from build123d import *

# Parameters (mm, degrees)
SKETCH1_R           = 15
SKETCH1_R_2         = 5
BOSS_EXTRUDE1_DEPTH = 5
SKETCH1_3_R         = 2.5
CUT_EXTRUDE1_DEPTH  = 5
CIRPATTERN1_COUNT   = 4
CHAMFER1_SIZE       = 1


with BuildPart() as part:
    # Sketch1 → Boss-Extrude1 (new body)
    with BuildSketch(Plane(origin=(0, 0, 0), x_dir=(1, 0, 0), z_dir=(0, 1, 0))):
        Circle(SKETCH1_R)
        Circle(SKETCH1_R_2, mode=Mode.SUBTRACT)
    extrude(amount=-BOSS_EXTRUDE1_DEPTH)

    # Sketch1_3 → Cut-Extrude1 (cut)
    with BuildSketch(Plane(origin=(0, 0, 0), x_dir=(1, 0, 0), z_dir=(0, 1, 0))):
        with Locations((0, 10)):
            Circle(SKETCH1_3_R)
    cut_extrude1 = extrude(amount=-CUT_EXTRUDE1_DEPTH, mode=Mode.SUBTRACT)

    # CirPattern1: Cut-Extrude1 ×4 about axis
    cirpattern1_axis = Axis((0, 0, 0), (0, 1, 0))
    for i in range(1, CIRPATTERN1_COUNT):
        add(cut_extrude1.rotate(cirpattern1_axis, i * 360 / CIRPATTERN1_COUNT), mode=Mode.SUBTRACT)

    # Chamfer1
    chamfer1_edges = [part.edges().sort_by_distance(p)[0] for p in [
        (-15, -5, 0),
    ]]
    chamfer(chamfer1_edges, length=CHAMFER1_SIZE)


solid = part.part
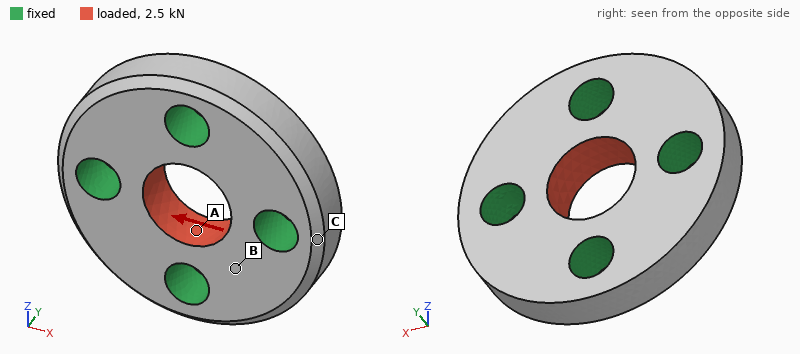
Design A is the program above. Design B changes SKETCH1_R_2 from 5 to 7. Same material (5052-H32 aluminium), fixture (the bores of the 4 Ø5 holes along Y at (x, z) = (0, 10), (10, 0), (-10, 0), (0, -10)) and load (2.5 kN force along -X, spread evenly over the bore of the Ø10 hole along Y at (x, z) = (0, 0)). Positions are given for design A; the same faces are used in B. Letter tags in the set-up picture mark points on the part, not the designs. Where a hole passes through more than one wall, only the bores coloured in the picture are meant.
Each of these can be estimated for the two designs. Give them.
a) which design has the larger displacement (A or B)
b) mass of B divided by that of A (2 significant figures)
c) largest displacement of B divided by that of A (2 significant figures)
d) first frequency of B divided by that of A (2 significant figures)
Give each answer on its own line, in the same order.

A
0.86
0.75
0.98
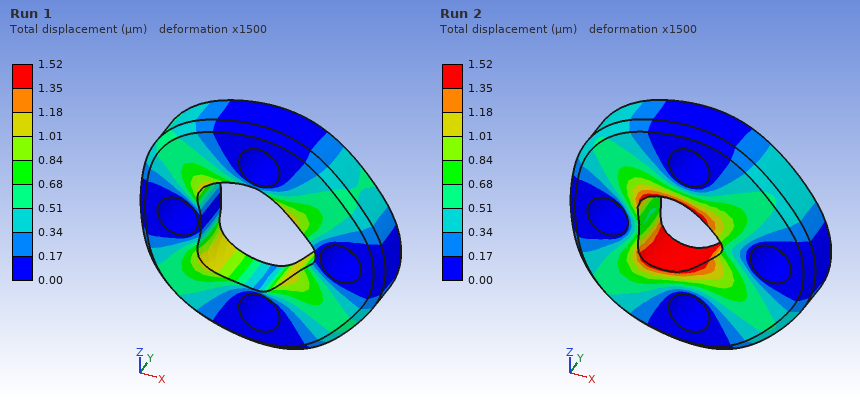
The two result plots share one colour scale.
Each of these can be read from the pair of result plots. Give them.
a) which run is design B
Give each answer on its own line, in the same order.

Run 1
